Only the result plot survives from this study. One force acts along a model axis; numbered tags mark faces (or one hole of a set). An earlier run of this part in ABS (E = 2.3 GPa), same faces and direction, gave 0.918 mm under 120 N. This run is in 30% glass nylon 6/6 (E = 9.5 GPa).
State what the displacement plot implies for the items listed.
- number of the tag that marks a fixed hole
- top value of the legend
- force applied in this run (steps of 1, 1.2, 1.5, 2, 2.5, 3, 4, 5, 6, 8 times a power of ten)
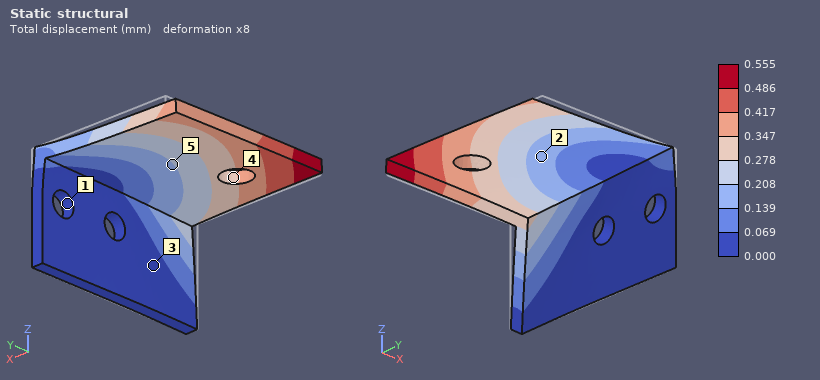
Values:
1
0.555 mm
300 N
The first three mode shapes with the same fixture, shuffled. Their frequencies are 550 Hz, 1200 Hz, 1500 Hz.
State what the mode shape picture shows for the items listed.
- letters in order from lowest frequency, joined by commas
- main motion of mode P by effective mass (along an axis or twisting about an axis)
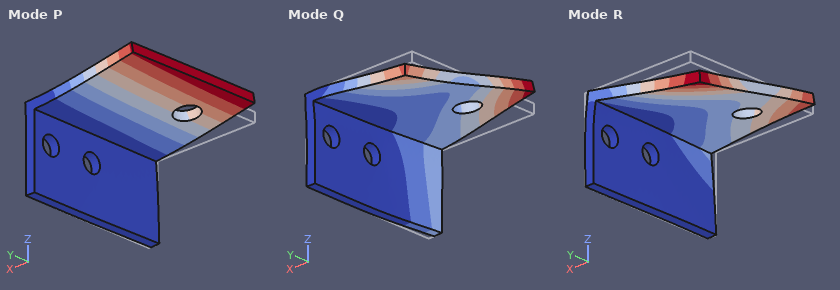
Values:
P, R, Q
along Z
